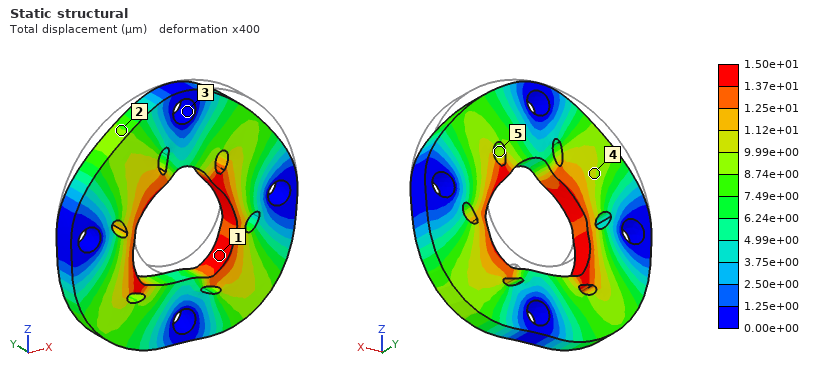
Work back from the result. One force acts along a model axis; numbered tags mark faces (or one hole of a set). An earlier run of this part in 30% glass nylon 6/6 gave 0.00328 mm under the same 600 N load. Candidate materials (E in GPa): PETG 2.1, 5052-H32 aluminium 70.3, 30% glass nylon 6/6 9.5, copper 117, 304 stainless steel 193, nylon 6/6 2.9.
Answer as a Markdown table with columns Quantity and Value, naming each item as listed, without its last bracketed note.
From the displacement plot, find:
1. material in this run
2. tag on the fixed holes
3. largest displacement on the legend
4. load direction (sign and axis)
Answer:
| Quantity | Value |
|---|---|
| material in this run | PETG |
| tag on the fixed holes | 3 |
| largest displacement on the legend | 1.50e+01 µm |
| load direction | -Z |
